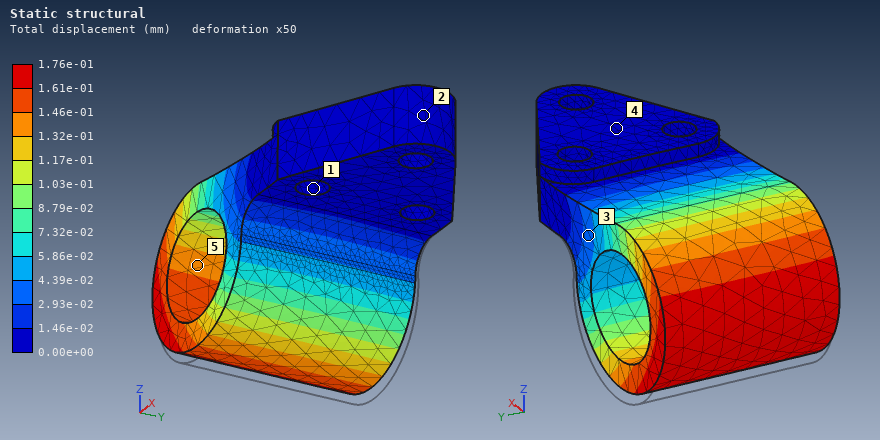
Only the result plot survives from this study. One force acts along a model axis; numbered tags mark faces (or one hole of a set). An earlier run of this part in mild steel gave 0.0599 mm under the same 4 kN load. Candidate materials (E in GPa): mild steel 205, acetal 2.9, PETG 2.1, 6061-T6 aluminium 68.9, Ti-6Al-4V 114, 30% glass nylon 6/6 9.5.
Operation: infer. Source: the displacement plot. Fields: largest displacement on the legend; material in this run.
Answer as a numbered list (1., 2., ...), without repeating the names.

1. 1.76e-01 mm
2. 6061-T6 aluminium
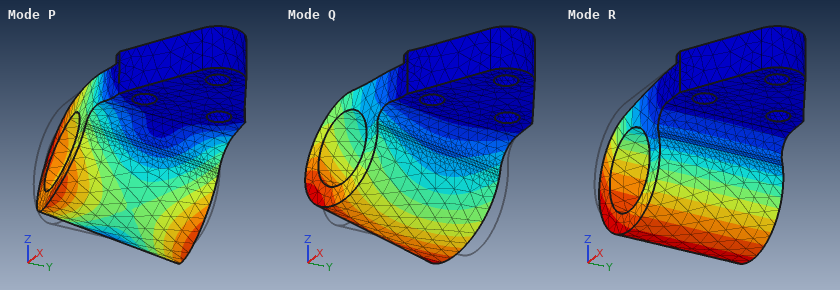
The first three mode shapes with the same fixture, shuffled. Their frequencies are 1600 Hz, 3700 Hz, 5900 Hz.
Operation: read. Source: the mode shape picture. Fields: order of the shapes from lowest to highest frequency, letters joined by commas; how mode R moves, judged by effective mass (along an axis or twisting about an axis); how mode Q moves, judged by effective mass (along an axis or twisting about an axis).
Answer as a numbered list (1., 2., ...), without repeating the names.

1. R, Q, P
2. along Z
3. along Y
